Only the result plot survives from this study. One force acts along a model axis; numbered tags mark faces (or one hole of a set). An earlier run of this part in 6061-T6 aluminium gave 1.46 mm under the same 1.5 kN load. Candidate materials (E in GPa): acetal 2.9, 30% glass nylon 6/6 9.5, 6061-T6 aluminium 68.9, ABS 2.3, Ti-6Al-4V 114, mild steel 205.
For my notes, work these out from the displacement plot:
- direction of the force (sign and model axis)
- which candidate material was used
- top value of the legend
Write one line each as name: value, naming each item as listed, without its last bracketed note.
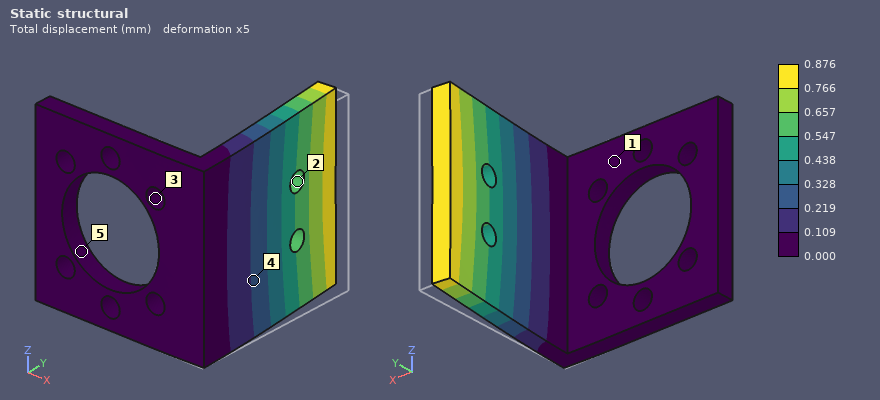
direction of the force: -X
which candidate material was used: Ti-6Al-4V
top value of the legend: 0.876 mm
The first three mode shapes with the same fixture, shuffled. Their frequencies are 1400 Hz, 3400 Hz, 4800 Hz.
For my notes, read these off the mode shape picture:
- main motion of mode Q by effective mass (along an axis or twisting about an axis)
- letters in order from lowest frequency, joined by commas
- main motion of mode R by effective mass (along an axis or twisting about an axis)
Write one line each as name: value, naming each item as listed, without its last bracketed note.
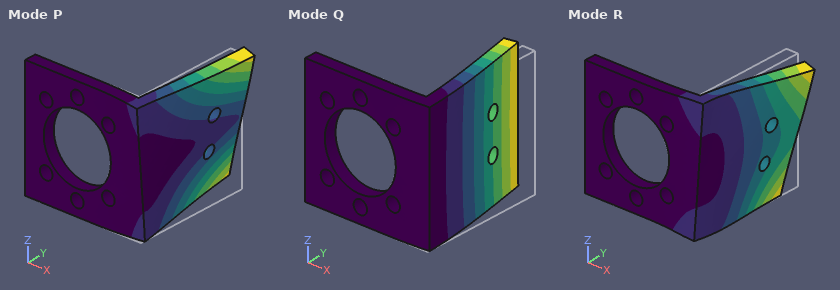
main motion of mode Q by effective mass: along X
letters in order from lowest frequency, joined by commas: Q, P, R
main motion of mode R by effective mass: along Z
